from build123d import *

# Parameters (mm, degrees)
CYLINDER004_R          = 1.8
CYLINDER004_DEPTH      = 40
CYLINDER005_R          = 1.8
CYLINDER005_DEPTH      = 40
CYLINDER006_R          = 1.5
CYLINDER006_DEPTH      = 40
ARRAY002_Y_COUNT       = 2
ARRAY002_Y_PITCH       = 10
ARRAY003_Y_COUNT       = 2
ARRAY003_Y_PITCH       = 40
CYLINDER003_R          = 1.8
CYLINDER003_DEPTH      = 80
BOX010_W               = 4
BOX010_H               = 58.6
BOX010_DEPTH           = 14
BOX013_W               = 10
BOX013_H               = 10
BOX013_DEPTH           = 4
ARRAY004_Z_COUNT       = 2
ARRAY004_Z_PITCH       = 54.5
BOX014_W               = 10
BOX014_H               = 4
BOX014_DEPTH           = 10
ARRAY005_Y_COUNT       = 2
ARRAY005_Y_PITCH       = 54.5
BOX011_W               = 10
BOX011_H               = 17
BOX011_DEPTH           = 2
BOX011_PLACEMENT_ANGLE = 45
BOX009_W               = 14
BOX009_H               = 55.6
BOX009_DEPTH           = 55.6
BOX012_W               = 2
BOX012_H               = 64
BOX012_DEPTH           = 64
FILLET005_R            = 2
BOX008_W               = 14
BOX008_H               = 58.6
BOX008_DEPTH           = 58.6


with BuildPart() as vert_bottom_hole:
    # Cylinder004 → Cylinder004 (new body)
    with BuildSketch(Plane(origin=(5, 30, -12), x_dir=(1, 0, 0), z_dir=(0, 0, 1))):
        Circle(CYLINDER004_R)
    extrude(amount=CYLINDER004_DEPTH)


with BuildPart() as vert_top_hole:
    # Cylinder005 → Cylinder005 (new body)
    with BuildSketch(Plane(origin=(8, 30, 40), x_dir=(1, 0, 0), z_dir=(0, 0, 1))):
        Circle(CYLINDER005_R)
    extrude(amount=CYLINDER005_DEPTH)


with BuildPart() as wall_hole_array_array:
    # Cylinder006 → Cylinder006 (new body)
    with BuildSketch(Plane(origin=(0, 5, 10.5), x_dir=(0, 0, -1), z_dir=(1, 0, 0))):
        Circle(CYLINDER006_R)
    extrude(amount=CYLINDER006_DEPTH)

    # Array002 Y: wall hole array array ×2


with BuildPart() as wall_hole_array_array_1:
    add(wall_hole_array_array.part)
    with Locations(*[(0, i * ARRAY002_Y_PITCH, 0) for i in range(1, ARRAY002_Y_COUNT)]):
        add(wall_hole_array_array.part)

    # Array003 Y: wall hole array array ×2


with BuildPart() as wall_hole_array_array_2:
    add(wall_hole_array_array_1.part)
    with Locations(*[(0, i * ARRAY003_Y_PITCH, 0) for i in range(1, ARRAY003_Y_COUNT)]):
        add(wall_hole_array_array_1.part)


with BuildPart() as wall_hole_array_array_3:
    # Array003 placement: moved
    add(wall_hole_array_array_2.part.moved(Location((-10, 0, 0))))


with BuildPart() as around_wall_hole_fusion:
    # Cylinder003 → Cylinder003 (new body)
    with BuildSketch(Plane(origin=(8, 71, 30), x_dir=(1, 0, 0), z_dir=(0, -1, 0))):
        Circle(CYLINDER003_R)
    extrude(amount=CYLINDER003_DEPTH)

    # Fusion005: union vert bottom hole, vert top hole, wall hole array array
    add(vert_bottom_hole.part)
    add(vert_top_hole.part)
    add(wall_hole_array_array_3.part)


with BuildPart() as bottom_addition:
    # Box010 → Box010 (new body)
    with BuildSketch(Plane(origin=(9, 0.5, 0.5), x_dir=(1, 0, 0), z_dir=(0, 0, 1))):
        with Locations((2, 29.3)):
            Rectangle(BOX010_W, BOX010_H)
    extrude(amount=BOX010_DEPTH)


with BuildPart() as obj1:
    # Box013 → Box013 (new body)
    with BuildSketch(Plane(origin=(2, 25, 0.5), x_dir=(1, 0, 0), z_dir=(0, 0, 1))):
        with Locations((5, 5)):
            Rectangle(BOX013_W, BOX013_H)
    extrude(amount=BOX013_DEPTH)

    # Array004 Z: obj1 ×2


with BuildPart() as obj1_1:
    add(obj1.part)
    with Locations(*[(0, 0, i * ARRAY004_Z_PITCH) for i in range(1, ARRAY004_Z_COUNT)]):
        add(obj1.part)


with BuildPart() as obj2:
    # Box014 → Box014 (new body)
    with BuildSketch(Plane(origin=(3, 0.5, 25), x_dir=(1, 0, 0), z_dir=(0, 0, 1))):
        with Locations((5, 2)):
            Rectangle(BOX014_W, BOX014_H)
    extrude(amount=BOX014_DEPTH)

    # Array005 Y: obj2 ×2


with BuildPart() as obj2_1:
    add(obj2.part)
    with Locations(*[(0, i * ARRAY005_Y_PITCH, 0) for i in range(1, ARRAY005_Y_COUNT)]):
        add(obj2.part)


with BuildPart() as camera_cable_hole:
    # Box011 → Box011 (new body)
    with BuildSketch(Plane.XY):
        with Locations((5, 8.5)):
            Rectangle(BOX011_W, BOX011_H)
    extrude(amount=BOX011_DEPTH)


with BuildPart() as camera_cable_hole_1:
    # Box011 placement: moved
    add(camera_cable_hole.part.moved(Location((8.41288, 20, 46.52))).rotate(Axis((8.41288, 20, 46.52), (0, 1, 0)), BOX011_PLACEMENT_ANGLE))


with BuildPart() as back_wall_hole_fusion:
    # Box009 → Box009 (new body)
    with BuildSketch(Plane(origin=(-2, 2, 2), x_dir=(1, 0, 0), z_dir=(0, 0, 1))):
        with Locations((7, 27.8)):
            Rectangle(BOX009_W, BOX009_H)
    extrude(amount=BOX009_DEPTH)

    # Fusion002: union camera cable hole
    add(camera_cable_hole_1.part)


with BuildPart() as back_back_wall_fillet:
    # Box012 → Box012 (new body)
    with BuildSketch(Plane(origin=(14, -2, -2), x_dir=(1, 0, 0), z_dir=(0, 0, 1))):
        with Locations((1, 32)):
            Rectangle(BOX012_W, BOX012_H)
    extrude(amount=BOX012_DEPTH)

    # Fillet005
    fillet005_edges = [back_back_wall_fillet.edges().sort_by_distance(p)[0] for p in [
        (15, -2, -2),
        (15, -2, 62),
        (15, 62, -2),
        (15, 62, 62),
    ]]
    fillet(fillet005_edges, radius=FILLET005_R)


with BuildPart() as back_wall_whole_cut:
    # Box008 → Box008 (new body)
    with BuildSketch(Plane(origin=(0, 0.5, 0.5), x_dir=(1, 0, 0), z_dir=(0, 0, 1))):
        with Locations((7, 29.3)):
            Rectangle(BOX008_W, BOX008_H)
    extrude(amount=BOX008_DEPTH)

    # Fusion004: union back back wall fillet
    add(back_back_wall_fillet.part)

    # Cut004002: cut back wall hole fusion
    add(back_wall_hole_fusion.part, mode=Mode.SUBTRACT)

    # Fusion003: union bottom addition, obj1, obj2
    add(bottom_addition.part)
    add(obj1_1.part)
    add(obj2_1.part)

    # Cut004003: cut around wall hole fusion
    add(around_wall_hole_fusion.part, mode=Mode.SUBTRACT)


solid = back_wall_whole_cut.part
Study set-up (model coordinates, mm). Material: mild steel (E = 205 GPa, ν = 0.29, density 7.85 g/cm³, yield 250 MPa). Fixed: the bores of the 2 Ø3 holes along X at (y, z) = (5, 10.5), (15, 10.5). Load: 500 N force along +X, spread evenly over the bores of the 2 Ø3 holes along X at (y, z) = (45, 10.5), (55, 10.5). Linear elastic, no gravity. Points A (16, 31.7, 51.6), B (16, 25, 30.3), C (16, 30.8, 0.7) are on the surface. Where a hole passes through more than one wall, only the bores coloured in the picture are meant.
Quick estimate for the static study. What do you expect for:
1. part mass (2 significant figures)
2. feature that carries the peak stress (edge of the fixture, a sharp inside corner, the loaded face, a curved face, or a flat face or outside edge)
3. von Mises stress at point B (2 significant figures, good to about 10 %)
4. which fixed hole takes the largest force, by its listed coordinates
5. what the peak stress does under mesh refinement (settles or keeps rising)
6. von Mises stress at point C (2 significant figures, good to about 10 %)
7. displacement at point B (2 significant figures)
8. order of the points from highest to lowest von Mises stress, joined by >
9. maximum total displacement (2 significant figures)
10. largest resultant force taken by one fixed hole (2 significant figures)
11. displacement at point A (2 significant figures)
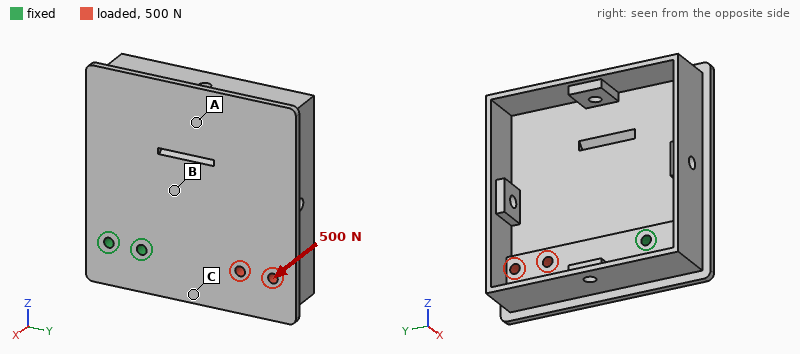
170 g
edge of the fixture
16 MPa
(15, 10.5)
keeps rising
29 MPa
11 µm
C > B > A
58 µm
1.2 kN
24 µm
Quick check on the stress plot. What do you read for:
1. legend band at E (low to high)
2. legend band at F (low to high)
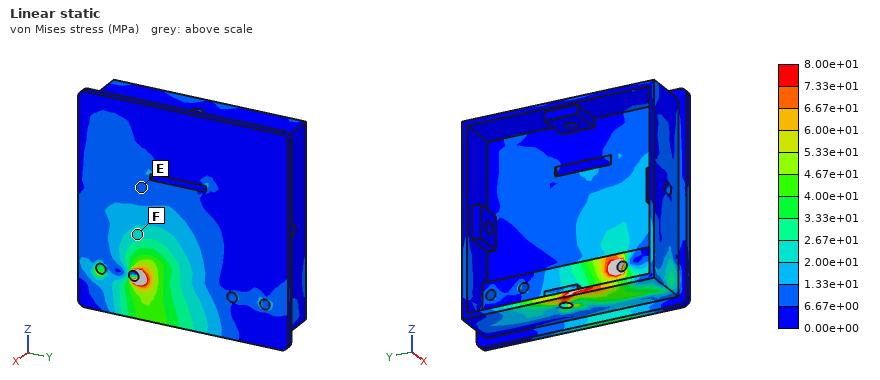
6.67e+00 to 1.33e+01 MPa
2.00e+01 to 2.67e+01 MPa
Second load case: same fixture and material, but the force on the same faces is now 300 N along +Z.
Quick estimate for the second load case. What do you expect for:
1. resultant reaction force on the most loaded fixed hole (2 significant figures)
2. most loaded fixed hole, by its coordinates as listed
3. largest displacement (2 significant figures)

1.1 kN
(15, 10.5)
11 µm
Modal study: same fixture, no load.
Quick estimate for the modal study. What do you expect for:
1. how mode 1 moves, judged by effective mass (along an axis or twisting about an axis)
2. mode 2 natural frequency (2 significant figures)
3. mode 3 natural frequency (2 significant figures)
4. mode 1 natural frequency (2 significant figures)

along X
2500 Hz
3200 Hz
1200 Hz
